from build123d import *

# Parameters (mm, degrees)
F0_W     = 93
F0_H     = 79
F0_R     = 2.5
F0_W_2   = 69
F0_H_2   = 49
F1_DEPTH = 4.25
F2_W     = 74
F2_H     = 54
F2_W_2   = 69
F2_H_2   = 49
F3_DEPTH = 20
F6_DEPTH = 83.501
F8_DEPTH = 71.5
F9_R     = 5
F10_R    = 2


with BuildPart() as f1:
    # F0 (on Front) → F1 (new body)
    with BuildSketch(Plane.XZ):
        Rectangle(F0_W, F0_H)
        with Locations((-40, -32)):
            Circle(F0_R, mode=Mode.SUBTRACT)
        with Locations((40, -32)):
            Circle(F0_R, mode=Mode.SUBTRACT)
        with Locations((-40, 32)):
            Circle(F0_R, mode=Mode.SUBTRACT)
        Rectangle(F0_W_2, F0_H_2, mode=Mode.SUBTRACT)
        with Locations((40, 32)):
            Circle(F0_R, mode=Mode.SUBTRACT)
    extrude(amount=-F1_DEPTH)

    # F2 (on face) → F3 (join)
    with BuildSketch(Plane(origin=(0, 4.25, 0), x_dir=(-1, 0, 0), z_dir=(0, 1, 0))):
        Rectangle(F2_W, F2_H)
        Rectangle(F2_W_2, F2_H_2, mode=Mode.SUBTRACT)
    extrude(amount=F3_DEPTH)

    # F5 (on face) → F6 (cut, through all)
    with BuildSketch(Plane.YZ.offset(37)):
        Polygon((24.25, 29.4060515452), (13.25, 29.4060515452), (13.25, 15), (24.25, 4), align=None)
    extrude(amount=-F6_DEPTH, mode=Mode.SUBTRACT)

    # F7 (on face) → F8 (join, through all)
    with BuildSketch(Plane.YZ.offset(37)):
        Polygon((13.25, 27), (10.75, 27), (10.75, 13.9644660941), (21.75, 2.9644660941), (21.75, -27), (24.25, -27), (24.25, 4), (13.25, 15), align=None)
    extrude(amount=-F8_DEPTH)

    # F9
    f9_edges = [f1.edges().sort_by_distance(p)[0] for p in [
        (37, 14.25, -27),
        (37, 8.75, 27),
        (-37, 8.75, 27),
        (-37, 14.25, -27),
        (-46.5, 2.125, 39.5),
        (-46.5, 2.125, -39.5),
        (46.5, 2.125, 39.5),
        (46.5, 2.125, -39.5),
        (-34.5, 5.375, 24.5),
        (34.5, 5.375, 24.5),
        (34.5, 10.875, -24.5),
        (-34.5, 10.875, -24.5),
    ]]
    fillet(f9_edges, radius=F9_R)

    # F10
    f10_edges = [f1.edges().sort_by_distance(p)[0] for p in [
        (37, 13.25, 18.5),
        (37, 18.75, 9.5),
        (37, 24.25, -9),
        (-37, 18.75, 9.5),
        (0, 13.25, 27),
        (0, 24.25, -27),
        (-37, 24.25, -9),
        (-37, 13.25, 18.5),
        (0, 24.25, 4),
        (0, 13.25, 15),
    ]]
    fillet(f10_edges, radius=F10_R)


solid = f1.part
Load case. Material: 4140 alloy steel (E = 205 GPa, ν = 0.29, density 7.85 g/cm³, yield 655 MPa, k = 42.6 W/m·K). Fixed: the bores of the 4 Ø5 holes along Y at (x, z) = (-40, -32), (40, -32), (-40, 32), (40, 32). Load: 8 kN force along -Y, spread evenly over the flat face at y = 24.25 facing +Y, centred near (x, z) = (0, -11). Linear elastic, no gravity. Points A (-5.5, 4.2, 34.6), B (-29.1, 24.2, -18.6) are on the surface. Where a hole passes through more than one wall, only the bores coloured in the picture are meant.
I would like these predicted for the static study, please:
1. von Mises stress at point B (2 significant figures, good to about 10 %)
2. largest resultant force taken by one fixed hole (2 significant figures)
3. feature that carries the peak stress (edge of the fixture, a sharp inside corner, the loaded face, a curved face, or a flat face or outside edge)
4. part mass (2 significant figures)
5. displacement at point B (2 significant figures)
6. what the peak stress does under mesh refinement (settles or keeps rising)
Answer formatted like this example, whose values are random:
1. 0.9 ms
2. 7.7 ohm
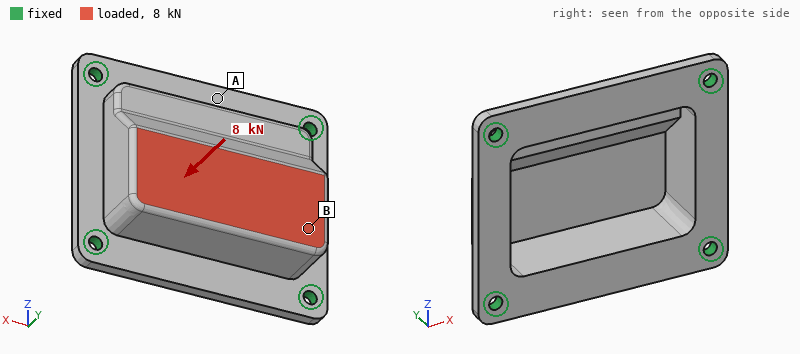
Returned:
1. 61 MPa
2. 3.3 kN
3. edge of the fixture
4. 270 g
5. 32 µm
6. keeps rising
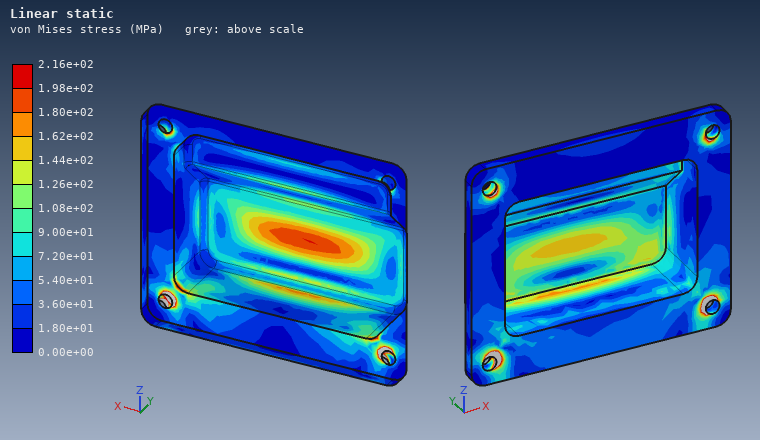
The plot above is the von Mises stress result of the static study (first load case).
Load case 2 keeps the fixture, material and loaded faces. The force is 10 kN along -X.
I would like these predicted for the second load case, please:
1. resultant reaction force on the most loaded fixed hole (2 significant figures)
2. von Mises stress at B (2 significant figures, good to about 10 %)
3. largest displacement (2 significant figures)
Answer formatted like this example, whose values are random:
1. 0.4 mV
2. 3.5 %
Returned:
1. 3.2 kN
2. 30 MPa
3. 24 µm
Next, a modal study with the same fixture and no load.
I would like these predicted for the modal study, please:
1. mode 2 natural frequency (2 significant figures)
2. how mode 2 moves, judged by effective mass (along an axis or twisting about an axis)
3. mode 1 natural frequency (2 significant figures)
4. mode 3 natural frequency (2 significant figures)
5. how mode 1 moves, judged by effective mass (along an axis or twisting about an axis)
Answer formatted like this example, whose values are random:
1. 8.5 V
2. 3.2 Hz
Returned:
1. 6400 Hz
2. along Y
3. 5000 Hz
4. 7100 Hz
5. along Y
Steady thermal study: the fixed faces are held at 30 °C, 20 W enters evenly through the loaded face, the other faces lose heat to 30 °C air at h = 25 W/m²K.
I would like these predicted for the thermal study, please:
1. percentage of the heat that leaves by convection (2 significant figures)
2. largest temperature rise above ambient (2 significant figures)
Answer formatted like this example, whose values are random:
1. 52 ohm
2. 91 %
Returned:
1. 40 %
2. 38 K
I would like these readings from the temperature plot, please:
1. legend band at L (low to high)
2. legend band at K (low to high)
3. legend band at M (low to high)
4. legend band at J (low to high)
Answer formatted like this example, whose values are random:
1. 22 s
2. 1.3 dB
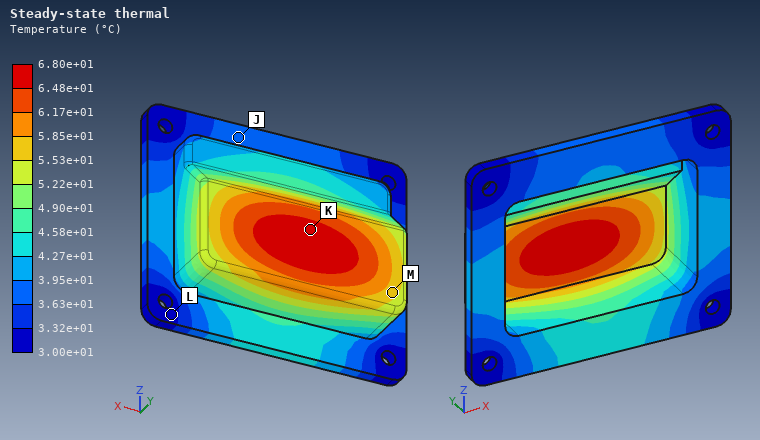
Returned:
1. 3.00e+01 to 3.32e+01 °C
2. 6.48e+01 to 6.80e+01 °C
3. 5.53e+01 to 5.85e+01 °C
4. 3.63e+01 to 3.95e+01 °C
